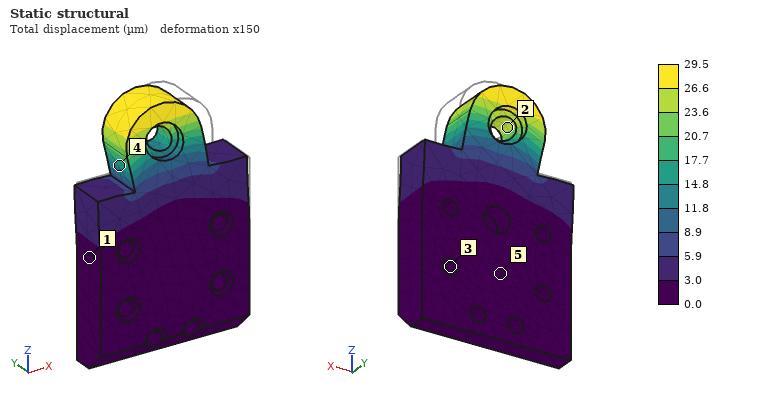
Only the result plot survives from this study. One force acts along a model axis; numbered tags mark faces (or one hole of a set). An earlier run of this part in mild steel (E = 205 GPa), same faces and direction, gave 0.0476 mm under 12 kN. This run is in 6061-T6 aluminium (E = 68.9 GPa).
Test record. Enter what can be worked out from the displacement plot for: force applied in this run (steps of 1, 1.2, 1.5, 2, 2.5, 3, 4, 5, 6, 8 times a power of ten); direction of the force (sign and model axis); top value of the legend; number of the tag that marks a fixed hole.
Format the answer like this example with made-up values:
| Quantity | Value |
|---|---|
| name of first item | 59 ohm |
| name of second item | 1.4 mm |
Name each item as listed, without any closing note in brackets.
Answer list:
| Quantity | Value |
|---|---|
| force applied in this run | 2.5 kN |
| direction of the force | -X |
| top value of the legend | 29.5 µm |
| number of the tag that marks a fixed hole | 3 |
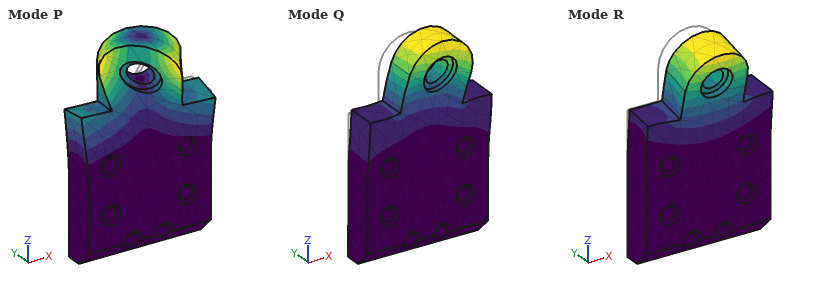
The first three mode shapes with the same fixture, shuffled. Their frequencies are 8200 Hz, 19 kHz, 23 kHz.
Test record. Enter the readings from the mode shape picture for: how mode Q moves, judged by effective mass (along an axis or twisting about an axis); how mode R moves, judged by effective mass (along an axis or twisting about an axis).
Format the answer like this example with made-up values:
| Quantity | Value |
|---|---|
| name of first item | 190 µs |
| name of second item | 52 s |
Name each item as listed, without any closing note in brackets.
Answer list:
| Quantity | Value |
|---|---|
| how mode Q moves, judged by effective mass | along X |
| how mode R moves, judged by effective mass | along Y |
